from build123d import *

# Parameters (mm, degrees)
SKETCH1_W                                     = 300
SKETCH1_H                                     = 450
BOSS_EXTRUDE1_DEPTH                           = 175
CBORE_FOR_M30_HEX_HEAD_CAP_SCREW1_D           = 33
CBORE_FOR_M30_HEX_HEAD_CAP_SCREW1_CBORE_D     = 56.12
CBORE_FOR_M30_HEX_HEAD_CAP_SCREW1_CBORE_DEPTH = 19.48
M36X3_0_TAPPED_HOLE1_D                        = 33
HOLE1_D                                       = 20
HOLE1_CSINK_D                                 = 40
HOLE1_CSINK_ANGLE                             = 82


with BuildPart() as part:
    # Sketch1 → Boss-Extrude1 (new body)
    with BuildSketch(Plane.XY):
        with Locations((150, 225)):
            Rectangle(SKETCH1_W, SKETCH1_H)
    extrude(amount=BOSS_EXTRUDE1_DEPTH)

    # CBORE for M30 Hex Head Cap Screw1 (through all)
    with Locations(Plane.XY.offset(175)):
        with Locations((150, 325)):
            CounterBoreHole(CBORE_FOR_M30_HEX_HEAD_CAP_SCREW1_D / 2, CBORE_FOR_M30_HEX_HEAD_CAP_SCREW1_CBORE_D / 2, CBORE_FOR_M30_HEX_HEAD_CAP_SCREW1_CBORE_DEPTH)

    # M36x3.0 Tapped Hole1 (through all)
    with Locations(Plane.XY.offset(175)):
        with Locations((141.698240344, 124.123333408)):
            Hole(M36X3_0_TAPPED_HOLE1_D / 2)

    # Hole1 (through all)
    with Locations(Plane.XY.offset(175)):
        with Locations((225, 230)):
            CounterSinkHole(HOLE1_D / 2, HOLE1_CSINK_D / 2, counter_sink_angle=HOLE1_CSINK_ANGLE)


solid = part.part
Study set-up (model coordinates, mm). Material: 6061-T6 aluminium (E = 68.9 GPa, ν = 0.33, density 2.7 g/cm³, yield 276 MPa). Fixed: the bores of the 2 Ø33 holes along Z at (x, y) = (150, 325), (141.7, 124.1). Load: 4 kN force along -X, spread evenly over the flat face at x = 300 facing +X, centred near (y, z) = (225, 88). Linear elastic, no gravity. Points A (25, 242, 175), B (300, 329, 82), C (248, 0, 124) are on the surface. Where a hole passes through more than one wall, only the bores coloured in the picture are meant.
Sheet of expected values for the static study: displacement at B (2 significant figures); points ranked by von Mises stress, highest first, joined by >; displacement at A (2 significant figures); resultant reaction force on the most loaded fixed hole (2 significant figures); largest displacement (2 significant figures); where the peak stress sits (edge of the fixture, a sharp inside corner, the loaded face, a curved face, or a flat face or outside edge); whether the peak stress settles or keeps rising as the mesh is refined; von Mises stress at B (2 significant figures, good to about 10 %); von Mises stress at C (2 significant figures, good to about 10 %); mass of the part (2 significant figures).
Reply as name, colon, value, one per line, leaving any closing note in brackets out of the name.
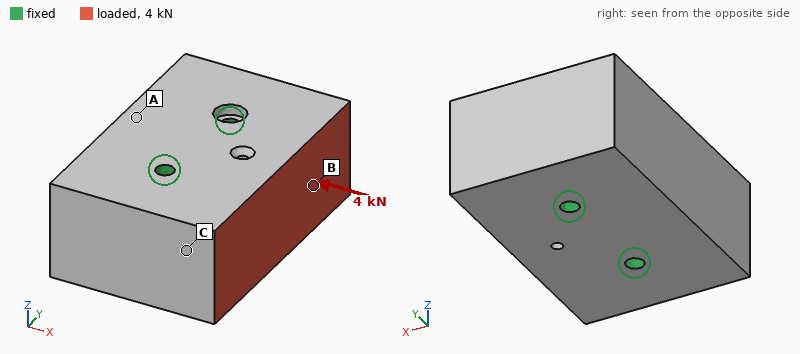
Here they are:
displacement at B: 0.17 µm
points ranked by von Mises stress, highest first, joined by >: B > C > A
displacement at A: 0.050 µm
resultant reaction force on the most loaded fixed hole: 2.0 kN
largest displacement: 0.27 µm
where the peak stress sits: edge of the fixture
whether the peak stress settles or keeps rising as the mesh is refined: keeps rising
von Mises stress at B: 0.069 MPa
von Mises stress at C: 0.045 MPa
mass of the part: 63 kg
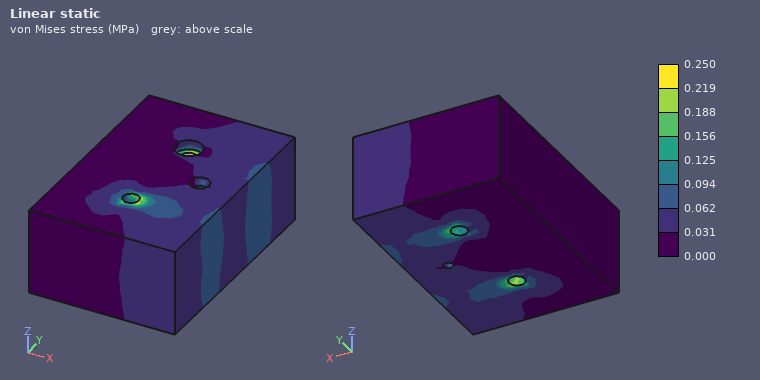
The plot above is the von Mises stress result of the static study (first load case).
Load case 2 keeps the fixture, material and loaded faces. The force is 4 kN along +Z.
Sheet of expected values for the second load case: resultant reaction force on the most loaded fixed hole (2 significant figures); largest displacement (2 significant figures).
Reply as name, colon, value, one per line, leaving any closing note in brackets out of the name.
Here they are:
resultant reaction force on the most loaded fixed hole: 2.0 kN
largest displacement: 1.4 µm
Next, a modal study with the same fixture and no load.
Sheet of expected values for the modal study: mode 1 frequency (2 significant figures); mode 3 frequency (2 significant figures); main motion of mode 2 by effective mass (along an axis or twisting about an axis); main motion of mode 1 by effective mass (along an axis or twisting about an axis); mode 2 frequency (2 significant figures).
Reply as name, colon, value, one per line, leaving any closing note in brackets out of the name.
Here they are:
mode 1 frequency: 2400 Hz
mode 3 frequency: 2800 Hz
main motion of mode 2 by effective mass: twisting about Z
main motion of mode 1 by effective mass: twisting about Y
mode 2 frequency: 2500 Hz
